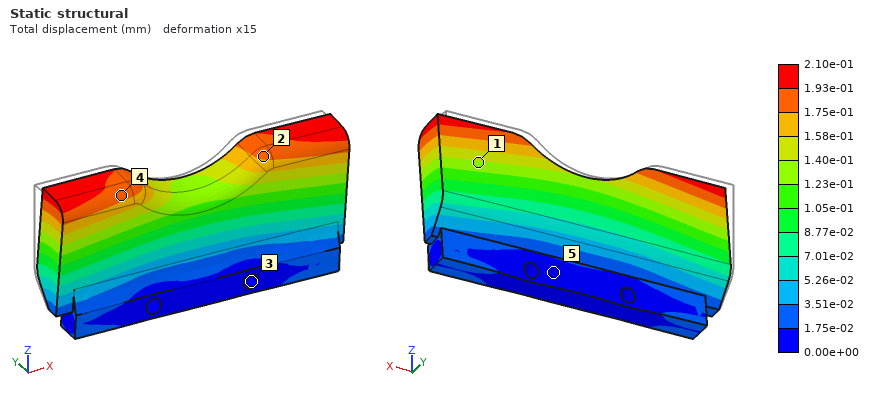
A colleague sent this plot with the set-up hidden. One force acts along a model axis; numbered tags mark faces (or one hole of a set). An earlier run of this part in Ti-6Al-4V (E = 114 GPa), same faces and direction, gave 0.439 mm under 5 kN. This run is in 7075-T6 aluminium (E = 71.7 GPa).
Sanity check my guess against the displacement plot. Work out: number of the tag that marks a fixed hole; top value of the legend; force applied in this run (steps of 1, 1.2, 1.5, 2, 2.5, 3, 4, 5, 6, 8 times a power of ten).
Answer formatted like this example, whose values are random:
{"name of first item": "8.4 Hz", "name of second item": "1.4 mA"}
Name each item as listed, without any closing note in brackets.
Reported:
{"number of the tag that marks a fixed hole": "3", "top value of the legend": "2.10e-01 mm", "force applied in this run": "1.5 kN"}
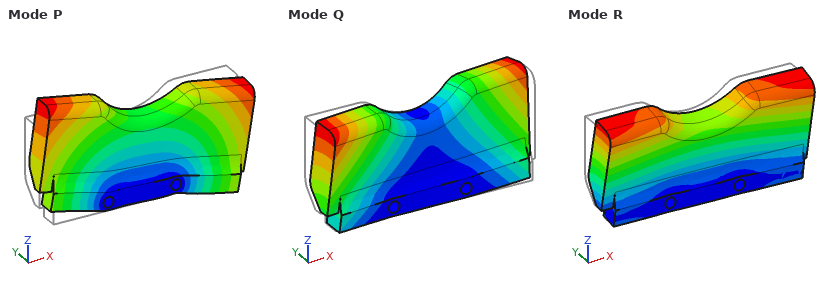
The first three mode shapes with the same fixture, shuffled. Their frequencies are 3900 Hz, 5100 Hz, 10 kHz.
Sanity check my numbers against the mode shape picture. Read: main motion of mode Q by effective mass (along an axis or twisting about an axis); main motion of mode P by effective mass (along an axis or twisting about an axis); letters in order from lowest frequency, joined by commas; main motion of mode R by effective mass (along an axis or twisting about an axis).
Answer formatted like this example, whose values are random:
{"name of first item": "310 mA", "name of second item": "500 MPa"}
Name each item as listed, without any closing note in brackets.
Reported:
{"main motion of mode Q by effective mass": "twisting about Z", "main motion of mode P by effective mass": "along X", "letters in order from lowest frequency, joined by commas": "R, Q, P", "main motion of mode R by effective mass": "along Y"}
